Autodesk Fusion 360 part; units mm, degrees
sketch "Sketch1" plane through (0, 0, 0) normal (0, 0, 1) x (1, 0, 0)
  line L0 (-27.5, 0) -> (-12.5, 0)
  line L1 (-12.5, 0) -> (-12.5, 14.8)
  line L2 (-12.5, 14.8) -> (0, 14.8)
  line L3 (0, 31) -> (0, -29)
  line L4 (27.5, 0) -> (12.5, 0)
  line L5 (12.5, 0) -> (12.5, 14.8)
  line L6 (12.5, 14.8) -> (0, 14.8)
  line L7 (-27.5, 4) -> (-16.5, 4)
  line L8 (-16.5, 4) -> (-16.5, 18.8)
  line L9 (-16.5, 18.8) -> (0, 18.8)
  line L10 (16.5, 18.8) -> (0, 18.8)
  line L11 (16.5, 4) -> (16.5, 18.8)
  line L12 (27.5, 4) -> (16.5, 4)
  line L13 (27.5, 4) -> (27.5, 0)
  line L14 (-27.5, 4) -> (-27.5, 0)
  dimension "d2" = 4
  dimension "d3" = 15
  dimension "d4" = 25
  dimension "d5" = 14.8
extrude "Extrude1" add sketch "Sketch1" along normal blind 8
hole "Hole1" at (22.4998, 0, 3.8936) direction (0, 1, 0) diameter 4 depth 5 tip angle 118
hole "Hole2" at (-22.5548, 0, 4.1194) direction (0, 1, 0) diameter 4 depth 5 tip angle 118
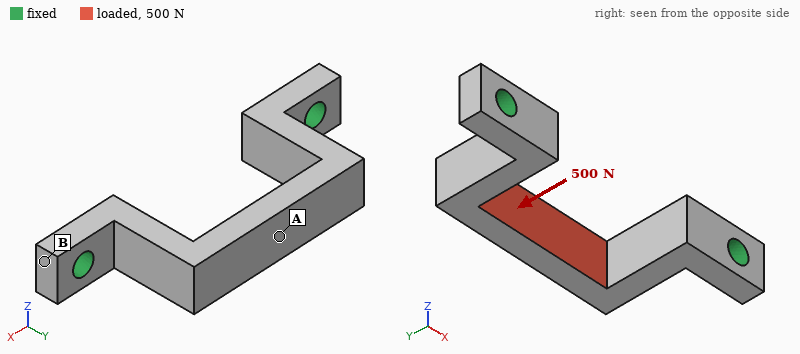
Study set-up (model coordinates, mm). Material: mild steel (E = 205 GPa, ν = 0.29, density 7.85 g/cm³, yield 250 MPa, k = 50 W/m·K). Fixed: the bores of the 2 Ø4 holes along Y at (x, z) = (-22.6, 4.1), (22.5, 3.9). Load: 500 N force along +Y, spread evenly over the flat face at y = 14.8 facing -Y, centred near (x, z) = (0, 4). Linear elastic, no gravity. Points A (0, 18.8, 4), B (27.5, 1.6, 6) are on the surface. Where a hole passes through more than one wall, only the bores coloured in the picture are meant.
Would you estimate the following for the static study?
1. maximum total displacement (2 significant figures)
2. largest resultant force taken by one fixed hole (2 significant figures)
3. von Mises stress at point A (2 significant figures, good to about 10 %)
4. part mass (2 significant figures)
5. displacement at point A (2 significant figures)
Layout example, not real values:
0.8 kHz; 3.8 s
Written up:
8.6 µm; 290 N; 43 MPa; 20 g; 8.3 µm
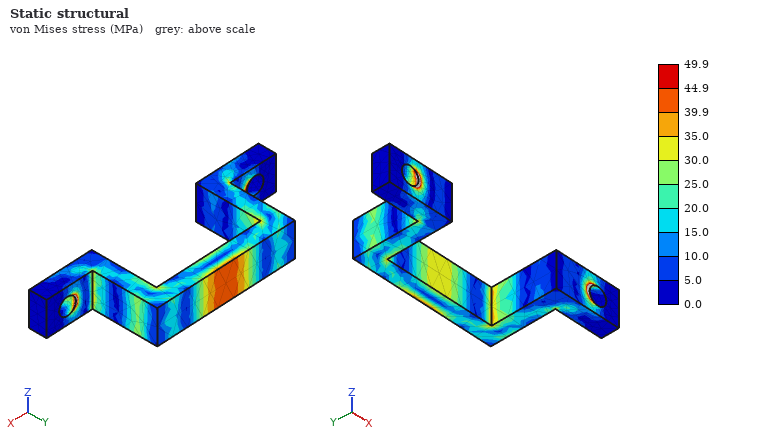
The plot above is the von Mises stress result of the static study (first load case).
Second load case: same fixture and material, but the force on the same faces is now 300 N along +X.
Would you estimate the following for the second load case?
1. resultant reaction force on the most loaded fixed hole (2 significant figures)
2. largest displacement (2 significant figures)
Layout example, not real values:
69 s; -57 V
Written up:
160 N; 12 µm
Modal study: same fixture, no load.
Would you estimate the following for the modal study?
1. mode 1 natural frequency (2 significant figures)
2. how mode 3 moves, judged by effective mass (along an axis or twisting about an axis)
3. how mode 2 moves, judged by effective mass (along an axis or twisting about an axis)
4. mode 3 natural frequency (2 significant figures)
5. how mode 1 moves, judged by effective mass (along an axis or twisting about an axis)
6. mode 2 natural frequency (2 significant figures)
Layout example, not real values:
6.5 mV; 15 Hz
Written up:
5600 Hz; twisting about Y; along X; 11 kHz; along Z; 8100 Hz
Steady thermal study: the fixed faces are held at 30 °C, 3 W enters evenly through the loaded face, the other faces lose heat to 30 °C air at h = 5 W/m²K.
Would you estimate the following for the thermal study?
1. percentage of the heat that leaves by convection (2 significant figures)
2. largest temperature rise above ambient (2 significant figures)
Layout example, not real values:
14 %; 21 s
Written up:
3.2 %; 24 K
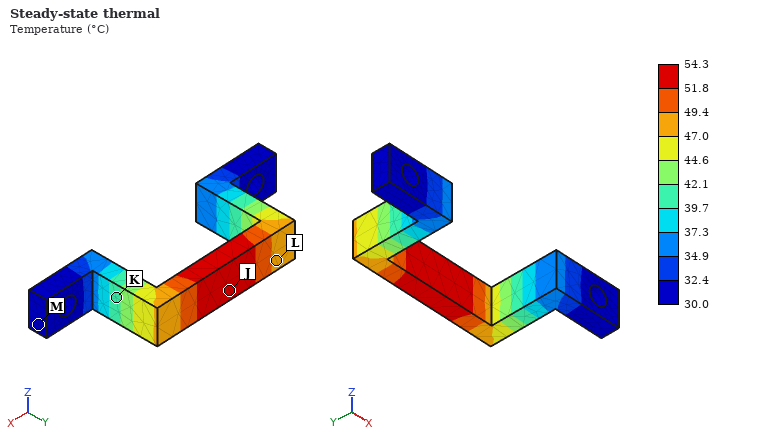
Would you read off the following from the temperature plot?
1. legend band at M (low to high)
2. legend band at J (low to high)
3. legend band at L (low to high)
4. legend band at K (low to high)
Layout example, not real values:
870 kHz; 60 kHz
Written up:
30.0 to 32.4 °C; 51.8 to 54.3 °C; 47.0 to 49.4 °C; 39.7 to 42.1 °C
